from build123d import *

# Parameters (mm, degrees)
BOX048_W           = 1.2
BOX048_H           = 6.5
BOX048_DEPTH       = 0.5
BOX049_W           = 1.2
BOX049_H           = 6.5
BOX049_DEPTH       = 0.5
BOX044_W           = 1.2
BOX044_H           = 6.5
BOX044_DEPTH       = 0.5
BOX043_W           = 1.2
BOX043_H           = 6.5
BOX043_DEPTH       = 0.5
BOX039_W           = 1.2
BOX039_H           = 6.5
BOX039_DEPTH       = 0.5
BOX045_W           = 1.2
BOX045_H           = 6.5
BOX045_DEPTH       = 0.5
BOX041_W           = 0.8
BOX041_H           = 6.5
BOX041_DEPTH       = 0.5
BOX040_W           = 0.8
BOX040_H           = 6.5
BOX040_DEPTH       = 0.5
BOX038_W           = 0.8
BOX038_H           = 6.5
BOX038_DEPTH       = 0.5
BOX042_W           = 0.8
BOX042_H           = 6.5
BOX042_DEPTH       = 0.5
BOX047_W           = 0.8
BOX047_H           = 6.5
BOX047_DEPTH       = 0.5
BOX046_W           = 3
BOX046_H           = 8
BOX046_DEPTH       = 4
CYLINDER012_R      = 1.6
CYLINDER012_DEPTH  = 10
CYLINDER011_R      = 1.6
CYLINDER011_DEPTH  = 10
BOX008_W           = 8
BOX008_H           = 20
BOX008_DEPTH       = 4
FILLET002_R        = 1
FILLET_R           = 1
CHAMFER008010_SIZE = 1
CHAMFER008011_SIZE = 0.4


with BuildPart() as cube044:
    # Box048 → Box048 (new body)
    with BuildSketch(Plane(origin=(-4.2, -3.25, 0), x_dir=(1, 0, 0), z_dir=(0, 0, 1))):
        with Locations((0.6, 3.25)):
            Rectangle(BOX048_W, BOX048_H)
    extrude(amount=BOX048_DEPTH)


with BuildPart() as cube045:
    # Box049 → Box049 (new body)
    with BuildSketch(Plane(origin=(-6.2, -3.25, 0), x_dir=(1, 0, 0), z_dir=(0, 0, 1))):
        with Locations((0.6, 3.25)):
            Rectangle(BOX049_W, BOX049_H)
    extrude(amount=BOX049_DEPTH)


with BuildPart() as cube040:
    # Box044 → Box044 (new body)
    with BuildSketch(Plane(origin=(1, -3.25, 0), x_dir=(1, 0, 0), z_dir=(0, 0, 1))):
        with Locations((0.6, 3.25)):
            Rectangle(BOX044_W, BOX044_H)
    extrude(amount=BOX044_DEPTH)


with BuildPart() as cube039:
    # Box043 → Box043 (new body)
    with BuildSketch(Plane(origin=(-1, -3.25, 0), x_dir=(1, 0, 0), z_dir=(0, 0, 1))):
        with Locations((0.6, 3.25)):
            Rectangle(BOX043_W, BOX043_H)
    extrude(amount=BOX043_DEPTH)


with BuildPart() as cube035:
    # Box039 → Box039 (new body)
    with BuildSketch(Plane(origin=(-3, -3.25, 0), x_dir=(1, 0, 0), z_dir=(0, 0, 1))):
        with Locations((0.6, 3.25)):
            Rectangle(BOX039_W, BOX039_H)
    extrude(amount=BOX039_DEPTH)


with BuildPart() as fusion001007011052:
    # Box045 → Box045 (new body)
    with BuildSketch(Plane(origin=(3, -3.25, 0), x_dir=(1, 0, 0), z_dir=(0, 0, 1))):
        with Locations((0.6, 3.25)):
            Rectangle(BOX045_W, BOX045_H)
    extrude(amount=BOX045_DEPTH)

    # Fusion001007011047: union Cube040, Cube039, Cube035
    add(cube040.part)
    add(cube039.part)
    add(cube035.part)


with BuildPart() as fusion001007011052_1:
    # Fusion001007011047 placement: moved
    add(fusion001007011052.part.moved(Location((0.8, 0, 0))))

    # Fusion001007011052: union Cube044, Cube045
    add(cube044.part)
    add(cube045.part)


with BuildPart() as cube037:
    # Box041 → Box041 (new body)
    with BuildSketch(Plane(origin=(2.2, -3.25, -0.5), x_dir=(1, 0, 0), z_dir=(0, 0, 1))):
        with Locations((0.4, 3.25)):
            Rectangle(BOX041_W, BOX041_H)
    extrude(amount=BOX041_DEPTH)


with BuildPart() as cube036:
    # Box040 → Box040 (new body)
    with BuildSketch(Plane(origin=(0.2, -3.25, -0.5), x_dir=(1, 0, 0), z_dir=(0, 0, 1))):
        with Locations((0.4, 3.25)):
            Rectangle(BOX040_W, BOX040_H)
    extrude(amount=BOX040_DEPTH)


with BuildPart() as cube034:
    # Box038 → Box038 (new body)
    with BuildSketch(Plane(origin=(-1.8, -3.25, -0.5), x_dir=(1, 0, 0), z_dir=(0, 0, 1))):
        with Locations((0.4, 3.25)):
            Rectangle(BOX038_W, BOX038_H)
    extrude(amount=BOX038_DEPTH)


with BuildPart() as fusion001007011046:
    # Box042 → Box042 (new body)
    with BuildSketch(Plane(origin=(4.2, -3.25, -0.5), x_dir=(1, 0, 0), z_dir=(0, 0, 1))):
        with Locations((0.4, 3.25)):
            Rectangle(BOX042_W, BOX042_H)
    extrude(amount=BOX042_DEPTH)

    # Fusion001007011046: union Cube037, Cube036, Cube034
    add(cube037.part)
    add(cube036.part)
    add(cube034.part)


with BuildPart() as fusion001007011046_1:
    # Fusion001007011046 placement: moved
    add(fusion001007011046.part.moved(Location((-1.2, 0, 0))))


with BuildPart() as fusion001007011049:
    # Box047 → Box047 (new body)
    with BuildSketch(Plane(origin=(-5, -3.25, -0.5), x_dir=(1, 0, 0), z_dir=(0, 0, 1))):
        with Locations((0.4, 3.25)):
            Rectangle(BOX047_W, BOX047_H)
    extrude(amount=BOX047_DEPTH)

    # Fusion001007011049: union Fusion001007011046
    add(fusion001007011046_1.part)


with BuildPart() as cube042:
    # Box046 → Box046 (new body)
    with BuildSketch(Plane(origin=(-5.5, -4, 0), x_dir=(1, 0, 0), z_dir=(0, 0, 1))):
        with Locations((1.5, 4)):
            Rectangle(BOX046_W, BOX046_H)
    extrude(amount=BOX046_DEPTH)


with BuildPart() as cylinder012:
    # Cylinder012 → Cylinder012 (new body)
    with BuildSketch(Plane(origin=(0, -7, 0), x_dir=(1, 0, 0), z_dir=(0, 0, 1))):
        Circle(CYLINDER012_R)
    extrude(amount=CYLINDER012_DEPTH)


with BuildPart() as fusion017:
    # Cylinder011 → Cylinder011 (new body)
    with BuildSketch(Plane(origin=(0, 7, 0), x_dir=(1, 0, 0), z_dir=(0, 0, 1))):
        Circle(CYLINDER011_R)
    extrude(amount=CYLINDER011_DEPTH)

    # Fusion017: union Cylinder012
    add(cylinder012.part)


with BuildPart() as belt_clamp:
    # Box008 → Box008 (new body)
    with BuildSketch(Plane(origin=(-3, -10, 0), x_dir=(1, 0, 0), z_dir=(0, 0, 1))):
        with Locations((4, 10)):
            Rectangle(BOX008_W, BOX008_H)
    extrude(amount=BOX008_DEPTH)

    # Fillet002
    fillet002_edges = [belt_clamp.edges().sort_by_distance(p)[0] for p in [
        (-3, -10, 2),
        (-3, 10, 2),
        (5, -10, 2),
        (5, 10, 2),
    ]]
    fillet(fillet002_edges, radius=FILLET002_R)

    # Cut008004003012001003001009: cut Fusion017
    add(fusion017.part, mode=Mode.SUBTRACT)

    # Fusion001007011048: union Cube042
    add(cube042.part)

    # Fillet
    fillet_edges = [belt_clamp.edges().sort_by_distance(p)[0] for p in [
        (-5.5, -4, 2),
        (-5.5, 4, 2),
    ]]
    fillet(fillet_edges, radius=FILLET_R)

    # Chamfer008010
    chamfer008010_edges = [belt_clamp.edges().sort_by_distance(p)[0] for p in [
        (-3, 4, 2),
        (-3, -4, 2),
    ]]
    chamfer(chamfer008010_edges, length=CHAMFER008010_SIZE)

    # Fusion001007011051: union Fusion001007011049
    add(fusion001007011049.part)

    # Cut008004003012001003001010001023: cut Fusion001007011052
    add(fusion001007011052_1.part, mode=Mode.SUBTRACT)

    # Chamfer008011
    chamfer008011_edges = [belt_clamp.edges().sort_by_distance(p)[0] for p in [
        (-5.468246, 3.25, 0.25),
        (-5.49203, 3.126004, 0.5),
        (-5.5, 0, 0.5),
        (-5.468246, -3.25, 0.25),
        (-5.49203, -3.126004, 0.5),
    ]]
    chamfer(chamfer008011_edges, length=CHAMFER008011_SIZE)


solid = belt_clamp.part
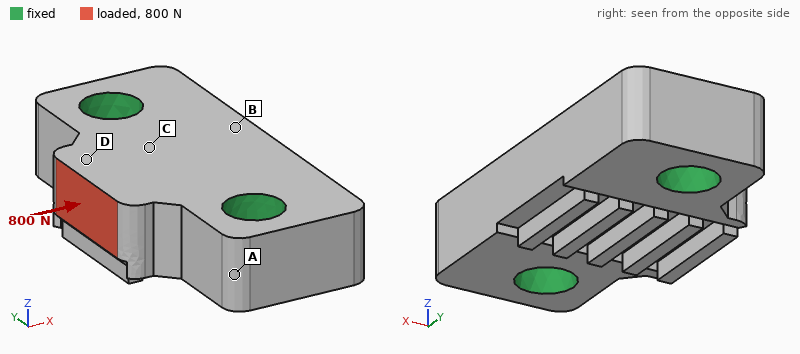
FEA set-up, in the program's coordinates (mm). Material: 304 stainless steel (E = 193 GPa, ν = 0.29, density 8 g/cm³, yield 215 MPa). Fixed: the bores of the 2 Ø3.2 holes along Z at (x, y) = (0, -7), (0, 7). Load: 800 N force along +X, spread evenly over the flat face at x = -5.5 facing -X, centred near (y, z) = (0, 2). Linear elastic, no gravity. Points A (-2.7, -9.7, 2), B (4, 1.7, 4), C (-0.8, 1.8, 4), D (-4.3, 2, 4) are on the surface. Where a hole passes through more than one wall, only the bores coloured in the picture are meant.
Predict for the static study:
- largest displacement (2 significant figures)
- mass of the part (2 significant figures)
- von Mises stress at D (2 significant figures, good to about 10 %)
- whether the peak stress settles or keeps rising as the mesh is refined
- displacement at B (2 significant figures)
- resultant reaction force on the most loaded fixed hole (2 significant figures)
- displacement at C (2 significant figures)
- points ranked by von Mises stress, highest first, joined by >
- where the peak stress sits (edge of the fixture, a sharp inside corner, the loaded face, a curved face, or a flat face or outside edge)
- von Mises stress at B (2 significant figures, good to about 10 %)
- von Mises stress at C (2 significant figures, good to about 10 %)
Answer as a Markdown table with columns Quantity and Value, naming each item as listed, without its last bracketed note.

| Quantity | Value |
|---|---|
| largest displacement | 2.2 µm |
| mass of the part | 5.2 g |
| von Mises stress at D | 41 MPa |
| whether the peak stress settles or keeps rising as the mesh is refined | keeps rising |
| displacement at B | 0.79 µm |
| resultant reaction force on the most loaded fixed hole | 410 N |
| displacement at C | 1.0 µm |
| points ranked by von Mises stress, highest first, joined by > | D > C > B > A |
| where the peak stress sits | edge of the fixture |
| von Mises stress at B | 12 MPa |
| von Mises stress at C | 26 MPa |
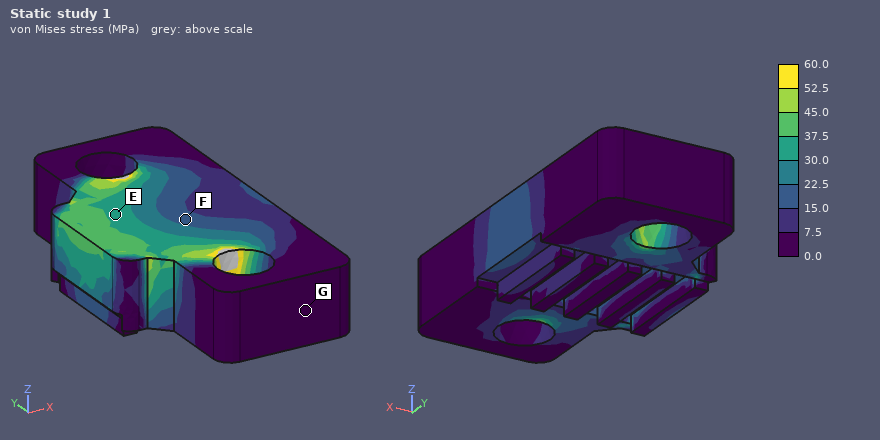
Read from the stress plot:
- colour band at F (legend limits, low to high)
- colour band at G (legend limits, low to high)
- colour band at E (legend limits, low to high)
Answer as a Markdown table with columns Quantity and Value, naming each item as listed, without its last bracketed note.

| Quantity | Value |
|---|---|
| colour band at F | 15.0 to 22.5 MPa |
| colour band at G | 0.0 to 7.5 MPa |
| colour band at E | 30.0 to 37.5 MPa |
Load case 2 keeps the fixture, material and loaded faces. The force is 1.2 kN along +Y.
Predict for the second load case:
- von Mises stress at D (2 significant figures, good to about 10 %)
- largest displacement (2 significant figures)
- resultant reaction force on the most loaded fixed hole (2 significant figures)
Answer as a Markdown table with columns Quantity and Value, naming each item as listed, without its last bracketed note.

| Quantity | Value |
|---|---|
| von Mises stress at D | 88 MPa |
| largest displacement | 3.2 µm |
| resultant reaction force on the most loaded fixed hole | 780 N |
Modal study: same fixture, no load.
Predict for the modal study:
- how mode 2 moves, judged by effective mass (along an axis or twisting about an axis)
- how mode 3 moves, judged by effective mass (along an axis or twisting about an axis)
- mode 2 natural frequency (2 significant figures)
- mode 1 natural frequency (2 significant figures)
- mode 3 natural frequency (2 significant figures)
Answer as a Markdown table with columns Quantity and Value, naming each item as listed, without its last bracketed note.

| Quantity | Value |
|---|---|
| how mode 2 moves, judged by effective mass | along Z |
| how mode 3 moves, judged by effective mass | along X |
| mode 2 natural frequency | 77 kHz |
| mode 1 natural frequency | 64 kHz |
| mode 3 natural frequency | 93 kHz |
